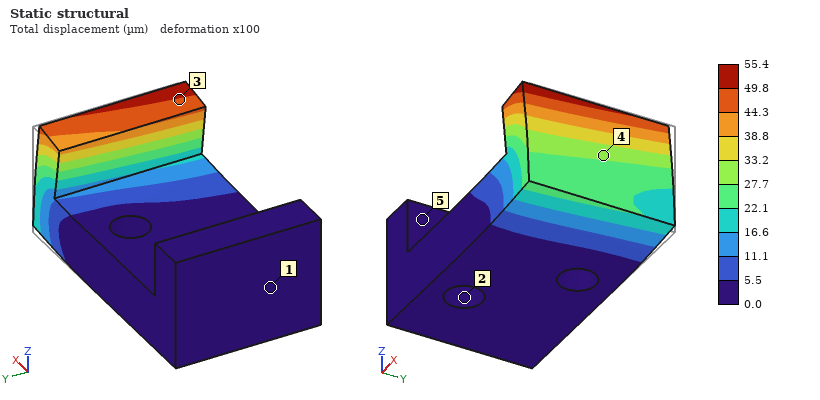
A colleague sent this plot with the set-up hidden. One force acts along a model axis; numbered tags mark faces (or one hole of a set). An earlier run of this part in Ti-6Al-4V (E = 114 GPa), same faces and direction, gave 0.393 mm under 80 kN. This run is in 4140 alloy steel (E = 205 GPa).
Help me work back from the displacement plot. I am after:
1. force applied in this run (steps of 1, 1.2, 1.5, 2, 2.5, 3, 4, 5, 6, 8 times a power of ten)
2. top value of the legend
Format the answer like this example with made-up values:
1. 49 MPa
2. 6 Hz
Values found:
1. 20 kN
2. 55.4 µm
